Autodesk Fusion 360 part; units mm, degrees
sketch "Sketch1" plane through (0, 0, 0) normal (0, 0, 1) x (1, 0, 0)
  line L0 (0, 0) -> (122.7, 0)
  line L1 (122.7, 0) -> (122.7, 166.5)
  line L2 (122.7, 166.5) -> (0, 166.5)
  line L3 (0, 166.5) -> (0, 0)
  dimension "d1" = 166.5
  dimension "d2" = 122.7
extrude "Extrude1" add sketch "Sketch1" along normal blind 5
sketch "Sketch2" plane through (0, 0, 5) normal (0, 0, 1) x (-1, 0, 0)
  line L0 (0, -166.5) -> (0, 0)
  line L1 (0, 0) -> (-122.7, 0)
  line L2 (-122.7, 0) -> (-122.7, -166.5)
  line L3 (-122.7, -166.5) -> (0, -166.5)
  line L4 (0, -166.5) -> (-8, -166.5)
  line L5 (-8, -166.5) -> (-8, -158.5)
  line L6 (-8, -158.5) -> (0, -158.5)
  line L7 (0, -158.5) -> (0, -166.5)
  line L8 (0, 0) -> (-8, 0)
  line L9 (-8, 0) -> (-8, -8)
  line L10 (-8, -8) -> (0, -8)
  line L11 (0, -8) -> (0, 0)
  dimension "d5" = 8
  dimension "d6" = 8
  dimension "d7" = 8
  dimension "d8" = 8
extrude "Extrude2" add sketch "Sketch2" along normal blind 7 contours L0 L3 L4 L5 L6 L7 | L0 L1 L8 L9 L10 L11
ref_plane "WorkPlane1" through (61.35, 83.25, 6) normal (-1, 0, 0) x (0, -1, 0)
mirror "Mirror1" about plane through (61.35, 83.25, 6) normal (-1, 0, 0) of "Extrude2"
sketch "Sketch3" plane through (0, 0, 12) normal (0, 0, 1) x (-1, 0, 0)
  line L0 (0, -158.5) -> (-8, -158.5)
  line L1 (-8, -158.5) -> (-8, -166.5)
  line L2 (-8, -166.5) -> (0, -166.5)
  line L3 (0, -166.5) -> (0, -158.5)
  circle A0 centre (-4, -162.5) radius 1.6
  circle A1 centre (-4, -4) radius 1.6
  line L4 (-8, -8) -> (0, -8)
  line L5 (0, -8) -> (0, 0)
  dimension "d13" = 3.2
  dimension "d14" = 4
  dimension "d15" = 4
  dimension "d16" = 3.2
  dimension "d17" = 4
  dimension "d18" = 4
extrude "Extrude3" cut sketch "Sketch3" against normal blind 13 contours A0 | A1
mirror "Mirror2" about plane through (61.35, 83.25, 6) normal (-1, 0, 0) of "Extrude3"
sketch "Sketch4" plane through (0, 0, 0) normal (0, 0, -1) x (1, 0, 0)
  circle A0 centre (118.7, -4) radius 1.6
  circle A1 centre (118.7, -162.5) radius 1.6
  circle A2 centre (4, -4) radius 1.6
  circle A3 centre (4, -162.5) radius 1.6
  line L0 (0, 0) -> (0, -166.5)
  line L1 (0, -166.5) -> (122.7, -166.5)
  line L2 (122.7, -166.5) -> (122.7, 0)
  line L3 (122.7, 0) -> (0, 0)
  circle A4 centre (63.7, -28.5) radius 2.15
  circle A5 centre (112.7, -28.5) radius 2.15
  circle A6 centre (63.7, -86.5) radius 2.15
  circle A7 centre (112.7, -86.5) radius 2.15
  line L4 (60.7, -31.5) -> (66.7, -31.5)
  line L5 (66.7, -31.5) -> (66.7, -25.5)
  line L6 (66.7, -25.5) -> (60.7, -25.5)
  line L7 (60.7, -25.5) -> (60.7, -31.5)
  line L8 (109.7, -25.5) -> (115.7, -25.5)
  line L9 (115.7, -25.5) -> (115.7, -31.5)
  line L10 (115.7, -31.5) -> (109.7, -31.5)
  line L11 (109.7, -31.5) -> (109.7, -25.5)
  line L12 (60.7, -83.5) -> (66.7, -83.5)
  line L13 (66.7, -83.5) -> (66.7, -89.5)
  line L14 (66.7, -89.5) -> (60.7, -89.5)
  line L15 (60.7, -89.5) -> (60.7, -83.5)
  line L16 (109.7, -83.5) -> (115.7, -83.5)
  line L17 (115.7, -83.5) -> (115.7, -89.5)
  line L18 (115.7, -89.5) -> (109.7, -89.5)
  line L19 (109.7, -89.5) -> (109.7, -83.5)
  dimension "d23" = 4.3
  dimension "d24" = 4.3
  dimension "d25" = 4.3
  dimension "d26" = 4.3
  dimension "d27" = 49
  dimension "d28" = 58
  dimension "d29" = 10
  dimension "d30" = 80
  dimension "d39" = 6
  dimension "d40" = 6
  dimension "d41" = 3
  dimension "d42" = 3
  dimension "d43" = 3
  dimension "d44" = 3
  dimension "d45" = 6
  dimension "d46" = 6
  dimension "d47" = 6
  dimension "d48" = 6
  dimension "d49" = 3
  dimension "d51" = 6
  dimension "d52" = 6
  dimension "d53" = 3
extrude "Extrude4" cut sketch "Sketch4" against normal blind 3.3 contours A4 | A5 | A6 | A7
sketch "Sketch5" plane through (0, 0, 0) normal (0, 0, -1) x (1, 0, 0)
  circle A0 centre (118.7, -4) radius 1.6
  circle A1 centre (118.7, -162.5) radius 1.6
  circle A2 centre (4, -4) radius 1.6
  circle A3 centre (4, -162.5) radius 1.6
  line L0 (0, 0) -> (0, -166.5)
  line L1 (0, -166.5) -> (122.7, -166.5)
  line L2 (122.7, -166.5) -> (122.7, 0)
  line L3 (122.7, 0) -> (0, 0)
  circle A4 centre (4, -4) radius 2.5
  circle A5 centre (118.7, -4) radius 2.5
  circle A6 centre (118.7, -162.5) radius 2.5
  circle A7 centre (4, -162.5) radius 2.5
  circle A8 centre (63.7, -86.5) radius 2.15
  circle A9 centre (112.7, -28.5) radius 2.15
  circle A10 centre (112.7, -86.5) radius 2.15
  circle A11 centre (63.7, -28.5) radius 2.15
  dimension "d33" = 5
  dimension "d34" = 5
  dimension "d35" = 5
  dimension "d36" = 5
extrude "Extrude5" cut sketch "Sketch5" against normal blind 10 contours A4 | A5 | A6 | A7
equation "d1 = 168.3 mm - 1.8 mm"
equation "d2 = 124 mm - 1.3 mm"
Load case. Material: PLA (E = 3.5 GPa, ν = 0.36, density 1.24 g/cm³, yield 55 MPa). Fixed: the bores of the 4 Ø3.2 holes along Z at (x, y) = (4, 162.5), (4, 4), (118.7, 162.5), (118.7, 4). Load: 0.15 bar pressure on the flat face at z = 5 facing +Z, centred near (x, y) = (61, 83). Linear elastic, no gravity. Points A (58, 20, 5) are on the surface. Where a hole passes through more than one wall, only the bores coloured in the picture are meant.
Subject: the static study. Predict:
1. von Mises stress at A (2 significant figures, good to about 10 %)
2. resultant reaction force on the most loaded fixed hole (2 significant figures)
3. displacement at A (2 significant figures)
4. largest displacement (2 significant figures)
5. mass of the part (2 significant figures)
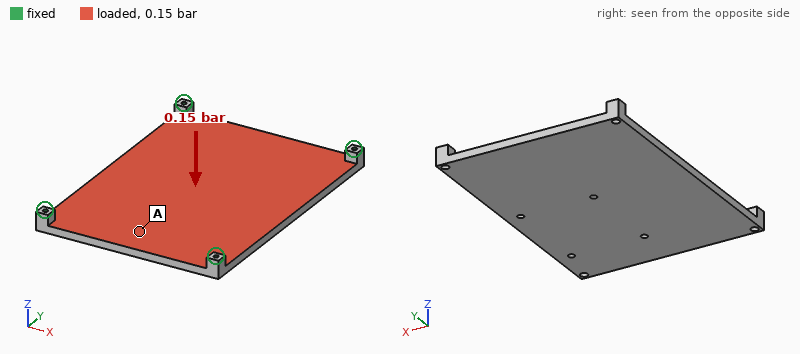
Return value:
3.2 MPa
170 N
0.76 mm
1.6 mm
130 g
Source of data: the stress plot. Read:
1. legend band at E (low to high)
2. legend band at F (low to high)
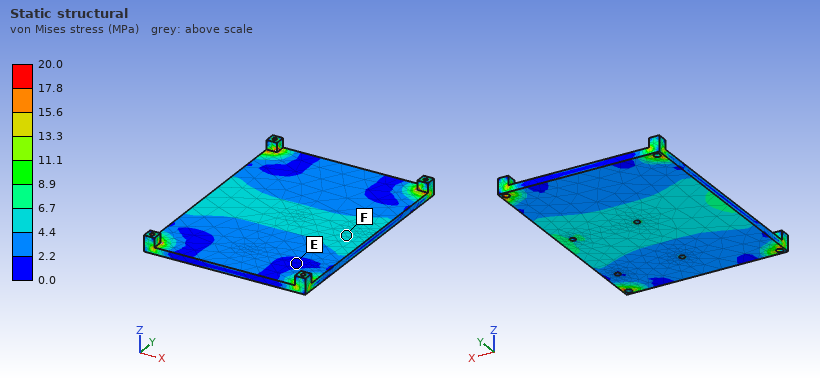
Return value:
0.0 to 2.2 MPa
4.4 to 6.7 MPa
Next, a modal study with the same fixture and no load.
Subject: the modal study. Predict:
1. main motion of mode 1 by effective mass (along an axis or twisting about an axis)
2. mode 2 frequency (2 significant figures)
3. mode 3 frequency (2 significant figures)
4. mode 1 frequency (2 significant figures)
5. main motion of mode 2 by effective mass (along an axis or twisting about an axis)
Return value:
along Z
390 Hz
500 Hz
220 Hz
twisting about Y
